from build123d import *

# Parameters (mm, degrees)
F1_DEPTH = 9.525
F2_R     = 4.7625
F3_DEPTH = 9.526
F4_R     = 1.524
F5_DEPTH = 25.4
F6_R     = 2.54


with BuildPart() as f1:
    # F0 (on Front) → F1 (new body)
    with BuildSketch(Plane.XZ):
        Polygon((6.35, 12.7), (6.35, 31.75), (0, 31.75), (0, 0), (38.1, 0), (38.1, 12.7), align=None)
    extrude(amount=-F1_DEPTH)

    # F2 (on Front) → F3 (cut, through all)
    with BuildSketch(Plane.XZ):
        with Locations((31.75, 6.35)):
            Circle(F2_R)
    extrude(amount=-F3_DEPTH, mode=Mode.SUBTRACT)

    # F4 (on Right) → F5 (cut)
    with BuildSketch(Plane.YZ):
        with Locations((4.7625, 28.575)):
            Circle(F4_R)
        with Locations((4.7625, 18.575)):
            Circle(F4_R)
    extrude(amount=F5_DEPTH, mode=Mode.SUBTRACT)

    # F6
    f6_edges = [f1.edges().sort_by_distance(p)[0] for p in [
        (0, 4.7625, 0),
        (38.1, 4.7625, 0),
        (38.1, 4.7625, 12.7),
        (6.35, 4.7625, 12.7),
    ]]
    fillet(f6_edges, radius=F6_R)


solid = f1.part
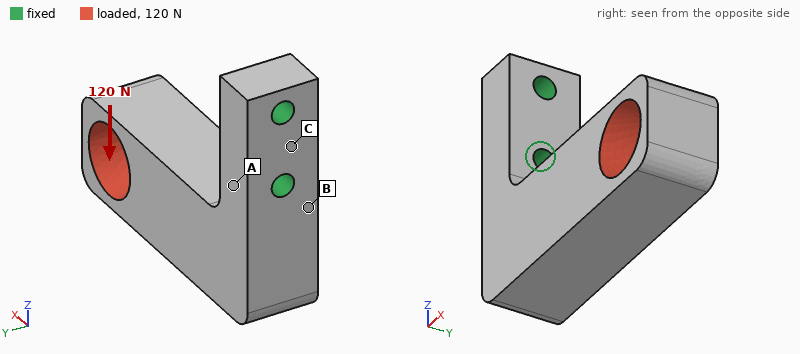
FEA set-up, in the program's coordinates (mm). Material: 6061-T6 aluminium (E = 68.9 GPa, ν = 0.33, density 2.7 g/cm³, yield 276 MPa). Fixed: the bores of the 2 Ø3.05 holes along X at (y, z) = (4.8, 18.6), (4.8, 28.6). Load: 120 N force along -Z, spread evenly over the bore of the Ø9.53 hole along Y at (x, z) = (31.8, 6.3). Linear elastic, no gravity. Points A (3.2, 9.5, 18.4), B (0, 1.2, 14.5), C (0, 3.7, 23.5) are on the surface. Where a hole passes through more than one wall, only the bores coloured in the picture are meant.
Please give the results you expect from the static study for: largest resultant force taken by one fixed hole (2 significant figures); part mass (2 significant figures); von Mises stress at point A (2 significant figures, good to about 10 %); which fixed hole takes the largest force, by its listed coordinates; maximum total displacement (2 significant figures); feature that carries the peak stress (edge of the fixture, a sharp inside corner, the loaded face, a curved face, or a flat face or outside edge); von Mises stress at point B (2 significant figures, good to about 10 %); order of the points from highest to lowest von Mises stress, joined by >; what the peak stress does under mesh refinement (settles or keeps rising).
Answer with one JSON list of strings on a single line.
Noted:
["120 N", "13 g", "17 MPa", "(4.8, 18.6)", "82 µm", "edge of the fixture", "42 MPa", "B > A > C", "keeps rising"]
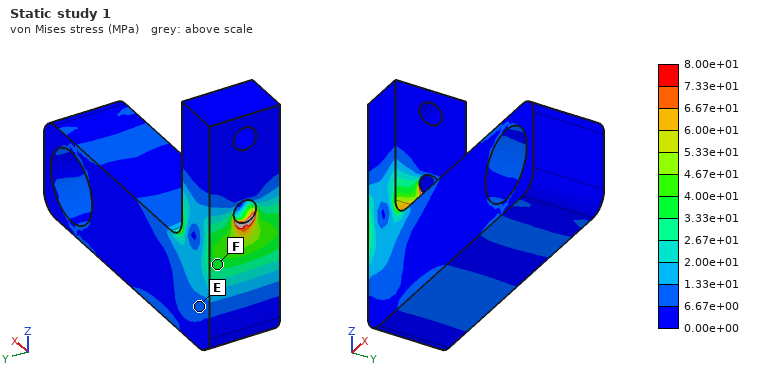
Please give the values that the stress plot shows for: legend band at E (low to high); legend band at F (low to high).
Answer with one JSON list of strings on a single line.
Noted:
["6.67e+00 to 1.33e+01 MPa", "3.33e+01 to 4.00e+01 MPa"]
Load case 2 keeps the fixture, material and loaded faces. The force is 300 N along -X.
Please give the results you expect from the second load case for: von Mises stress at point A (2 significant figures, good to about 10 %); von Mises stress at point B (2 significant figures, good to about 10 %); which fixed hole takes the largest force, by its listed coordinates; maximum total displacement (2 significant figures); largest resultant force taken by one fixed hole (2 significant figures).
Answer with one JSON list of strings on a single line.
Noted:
["10 MPa", "31 MPa", "(4.8, 18.6)", "52 µm", "350 N"]
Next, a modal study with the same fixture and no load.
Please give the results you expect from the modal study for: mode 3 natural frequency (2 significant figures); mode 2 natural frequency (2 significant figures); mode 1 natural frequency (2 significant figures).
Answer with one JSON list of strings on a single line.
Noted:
["10 kHz", "3400 Hz", "3300 Hz"]
